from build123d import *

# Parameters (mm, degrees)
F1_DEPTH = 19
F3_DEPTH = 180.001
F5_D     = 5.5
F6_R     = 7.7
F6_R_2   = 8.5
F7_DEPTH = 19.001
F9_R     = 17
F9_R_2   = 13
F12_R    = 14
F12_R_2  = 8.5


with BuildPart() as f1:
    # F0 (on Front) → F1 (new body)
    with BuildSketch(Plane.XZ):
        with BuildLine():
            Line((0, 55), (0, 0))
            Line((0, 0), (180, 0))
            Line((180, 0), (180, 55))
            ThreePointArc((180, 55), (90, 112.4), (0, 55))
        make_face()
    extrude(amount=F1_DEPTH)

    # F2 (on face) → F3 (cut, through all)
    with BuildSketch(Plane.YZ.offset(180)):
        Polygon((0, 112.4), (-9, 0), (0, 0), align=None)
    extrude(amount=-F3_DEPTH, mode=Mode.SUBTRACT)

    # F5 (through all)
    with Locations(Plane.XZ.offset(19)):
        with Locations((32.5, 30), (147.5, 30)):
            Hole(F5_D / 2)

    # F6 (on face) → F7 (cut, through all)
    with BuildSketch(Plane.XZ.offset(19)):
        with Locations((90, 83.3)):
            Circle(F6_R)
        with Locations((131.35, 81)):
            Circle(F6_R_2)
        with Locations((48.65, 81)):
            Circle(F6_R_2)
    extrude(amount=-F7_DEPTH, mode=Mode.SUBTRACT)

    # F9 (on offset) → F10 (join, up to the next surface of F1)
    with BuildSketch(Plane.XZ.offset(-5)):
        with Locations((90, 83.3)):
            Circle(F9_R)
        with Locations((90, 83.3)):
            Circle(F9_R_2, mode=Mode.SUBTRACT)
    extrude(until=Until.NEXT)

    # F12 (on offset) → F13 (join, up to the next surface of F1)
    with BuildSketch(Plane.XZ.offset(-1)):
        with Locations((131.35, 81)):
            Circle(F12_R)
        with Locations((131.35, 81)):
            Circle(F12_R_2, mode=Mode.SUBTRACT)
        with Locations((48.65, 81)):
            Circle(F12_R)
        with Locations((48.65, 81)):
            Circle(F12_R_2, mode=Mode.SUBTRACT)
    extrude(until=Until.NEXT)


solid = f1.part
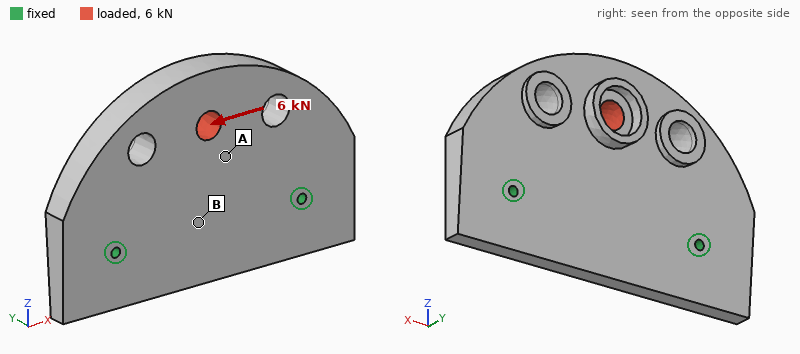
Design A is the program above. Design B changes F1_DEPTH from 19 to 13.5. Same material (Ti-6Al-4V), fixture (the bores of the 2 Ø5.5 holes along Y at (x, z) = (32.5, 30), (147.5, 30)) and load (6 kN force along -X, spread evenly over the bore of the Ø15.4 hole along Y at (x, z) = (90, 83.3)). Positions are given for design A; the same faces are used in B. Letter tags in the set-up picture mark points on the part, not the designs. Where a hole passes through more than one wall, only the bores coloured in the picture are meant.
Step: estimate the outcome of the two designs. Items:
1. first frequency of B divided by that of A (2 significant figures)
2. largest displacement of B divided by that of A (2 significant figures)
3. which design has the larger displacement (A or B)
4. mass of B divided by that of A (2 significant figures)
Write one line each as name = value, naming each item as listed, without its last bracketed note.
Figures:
first frequency of B divided by that of A = 0.59
largest displacement of B divided by that of A = 1.7
which design has the larger displacement = B
mass of B divided by that of A = 0.61
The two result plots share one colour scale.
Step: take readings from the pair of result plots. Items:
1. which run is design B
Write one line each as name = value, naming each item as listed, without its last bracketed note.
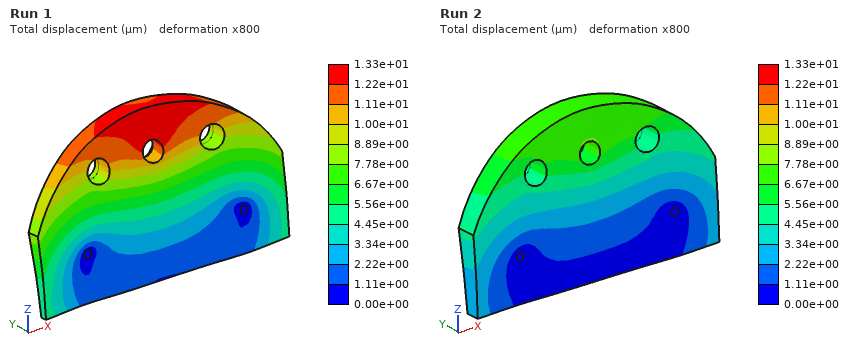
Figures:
which run is design B = Run 1
